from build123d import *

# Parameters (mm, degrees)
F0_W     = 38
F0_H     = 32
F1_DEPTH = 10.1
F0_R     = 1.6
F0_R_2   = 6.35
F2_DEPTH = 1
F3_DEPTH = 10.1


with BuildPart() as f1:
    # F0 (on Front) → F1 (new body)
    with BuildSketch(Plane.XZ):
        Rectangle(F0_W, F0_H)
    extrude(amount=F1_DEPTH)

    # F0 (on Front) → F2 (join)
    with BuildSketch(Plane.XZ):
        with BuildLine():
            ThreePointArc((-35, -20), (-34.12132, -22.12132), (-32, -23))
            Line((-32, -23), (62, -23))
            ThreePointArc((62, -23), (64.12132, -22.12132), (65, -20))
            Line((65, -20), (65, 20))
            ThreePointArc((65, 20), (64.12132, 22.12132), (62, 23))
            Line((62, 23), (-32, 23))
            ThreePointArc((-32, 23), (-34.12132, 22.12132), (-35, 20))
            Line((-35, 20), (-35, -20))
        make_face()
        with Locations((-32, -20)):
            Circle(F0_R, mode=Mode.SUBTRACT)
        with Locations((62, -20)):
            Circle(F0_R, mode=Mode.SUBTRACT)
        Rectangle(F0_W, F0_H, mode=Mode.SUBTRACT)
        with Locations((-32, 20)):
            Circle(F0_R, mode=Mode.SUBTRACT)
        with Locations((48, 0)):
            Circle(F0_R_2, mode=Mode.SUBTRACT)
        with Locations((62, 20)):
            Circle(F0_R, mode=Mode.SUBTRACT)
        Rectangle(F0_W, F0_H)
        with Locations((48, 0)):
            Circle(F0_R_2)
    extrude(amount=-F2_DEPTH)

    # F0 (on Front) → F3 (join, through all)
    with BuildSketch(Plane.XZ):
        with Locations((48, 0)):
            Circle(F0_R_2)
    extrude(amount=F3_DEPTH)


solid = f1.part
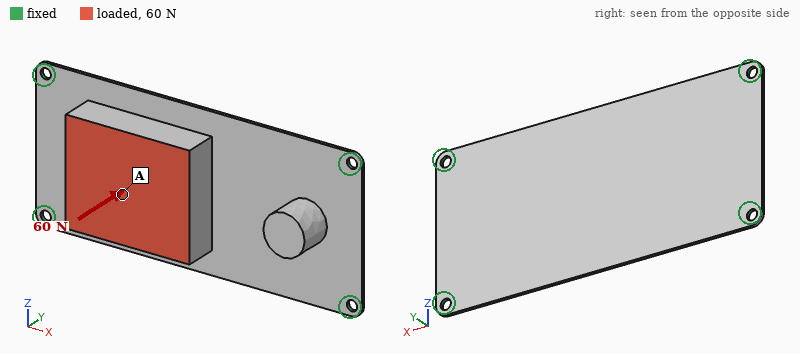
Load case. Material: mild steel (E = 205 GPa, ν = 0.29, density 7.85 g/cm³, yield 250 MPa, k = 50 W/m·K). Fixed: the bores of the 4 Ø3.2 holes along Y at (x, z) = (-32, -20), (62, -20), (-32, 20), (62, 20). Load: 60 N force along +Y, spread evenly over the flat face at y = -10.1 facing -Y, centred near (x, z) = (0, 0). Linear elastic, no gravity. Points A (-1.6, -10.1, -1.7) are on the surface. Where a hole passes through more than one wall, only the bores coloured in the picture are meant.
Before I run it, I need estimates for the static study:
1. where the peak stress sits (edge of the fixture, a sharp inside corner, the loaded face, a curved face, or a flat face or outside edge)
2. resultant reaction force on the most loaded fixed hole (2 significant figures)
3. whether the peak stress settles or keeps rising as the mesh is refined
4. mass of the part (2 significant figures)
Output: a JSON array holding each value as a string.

["edge of the fixture", "23 N", "keeps rising", "140 g"]
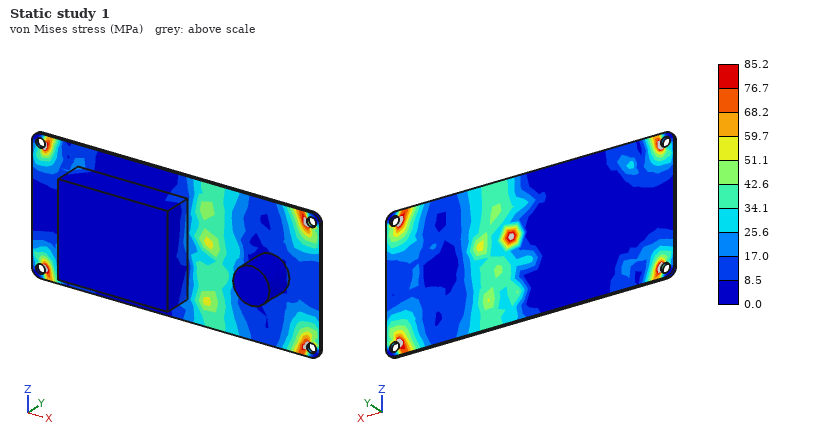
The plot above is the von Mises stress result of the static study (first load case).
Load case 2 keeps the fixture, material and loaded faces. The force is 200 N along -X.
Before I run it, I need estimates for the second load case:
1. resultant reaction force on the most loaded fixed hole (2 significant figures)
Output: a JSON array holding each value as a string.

["64 N"]
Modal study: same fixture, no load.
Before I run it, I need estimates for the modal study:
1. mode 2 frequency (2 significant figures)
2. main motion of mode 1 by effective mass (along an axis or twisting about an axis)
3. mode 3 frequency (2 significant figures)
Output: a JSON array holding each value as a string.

["1100 Hz", "along Y", "1500 Hz"]
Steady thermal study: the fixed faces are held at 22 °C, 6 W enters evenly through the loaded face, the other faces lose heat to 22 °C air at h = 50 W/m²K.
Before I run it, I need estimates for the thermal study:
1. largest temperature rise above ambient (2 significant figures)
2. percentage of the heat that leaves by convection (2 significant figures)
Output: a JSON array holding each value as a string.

["16 K", "75 %"]
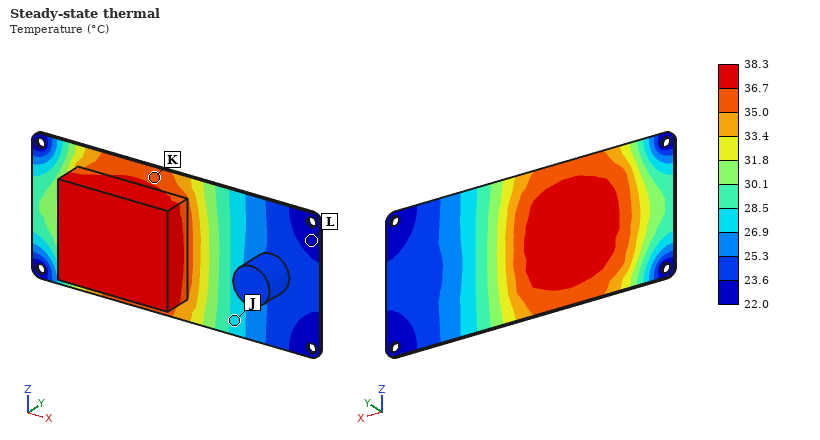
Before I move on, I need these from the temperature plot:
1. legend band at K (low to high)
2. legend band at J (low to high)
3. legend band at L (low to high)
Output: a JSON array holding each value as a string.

["35.0 to 36.7 °C", "26.9 to 28.5 °C", "22.0 to 23.6 °C"]
